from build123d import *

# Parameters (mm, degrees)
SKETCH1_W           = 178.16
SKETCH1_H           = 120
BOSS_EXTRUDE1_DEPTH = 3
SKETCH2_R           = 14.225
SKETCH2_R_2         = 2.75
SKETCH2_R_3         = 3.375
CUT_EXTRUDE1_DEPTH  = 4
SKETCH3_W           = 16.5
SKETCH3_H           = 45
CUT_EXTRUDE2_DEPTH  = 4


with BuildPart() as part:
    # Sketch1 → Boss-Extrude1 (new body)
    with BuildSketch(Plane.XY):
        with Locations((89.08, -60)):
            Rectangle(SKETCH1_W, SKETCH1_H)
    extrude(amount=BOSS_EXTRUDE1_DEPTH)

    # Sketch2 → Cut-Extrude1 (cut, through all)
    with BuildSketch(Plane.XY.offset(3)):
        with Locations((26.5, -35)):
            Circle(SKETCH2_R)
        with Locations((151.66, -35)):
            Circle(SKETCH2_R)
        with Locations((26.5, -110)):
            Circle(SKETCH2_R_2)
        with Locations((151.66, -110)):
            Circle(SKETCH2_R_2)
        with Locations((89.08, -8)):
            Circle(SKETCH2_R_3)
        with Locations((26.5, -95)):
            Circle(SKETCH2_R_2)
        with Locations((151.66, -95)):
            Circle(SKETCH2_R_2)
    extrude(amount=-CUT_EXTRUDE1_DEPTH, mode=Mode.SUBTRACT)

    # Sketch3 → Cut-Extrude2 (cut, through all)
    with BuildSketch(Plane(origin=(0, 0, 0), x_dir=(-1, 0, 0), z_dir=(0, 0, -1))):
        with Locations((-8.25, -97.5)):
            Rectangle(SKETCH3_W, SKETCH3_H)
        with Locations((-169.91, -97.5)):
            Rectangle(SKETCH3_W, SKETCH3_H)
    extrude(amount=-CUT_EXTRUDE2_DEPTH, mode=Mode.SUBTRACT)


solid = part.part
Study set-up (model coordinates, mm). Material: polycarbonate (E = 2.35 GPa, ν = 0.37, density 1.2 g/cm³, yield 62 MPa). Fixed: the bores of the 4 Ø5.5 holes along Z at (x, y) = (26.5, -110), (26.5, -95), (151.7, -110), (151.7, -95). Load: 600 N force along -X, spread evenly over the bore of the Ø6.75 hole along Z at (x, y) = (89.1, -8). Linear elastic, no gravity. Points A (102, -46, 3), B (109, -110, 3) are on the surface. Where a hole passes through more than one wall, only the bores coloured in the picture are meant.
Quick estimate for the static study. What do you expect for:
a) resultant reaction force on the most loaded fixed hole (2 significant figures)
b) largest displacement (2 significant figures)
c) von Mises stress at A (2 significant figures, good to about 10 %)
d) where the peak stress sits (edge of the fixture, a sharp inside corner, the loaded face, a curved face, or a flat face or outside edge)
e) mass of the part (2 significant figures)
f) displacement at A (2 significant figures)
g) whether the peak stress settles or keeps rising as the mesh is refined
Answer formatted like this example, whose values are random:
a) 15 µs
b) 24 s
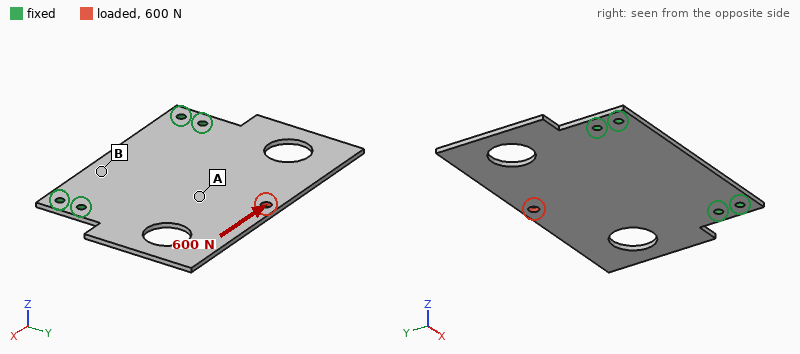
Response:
a) 380 N
b) 0.35 mm
c) 3.2 MPa
d) edge of the fixture
e) 67 g
f) 0.15 mm
g) keeps rising
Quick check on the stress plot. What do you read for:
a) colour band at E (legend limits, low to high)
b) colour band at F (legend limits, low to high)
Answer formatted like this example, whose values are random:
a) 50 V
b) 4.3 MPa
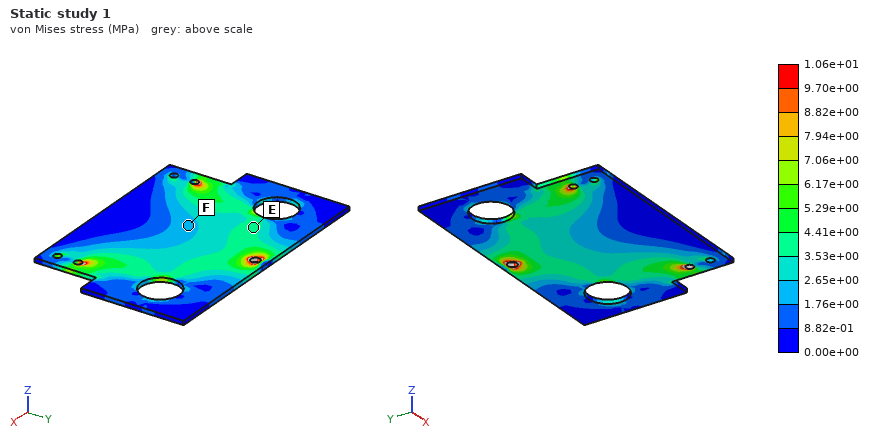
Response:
a) 3.53e+00 to 4.41e+00 MPa
b) 1.76e+00 to 2.65e+00 MPa
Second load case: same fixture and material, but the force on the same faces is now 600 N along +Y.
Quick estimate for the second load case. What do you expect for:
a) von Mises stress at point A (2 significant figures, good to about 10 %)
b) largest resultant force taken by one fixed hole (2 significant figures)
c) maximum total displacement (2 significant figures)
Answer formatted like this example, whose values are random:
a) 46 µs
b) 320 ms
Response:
a) 2.6 MPa
b) 210 N
c) 0.23 mm
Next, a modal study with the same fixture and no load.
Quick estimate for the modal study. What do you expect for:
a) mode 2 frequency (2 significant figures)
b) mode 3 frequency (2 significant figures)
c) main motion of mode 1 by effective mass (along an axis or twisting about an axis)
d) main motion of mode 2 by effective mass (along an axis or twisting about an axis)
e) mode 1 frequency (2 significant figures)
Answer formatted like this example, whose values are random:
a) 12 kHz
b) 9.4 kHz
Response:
a) 110 Hz
b) 190 Hz
c) along Z
d) twisting about Y
e) 61 Hz
